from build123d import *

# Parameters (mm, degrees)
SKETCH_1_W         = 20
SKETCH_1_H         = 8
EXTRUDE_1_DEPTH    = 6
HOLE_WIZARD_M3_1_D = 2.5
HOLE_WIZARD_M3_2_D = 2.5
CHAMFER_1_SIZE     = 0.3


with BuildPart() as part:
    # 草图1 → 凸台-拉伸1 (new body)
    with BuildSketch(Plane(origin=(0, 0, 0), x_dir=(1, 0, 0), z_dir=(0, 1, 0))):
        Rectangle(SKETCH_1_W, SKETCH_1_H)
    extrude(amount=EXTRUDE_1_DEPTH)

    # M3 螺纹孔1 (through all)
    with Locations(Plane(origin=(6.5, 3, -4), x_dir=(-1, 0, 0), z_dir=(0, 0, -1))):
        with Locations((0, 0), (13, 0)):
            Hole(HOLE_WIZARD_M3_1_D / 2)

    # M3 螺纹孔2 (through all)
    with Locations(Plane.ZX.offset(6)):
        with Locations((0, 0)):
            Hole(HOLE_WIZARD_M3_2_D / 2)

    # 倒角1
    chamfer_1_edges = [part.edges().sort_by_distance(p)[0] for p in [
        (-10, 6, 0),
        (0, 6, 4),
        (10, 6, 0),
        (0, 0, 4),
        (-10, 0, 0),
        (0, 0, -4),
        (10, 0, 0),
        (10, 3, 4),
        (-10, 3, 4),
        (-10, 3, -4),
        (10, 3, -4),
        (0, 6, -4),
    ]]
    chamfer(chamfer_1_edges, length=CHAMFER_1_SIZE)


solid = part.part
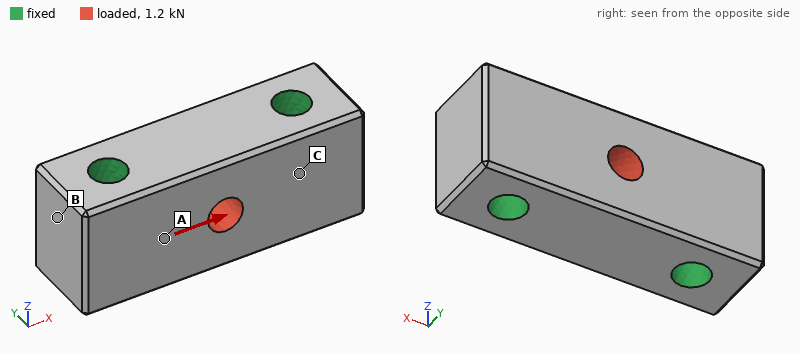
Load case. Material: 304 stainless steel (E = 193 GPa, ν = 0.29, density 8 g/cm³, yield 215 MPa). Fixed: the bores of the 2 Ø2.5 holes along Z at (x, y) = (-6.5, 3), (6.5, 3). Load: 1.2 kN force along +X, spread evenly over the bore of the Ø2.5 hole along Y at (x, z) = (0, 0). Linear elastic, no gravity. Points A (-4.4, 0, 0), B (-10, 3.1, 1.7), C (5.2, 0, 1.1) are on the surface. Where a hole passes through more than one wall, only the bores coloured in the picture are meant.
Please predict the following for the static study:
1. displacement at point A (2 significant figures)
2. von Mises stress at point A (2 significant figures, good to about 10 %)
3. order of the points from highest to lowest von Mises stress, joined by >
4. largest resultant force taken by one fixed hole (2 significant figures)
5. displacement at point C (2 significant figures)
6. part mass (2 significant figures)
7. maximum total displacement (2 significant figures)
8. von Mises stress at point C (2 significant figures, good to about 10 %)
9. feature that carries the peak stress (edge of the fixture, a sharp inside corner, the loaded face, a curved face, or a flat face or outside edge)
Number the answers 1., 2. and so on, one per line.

1. 0.19 µm
2. 12 MPa
3. A > C > B
4. 600 N
5. 0.14 µm
6. 6.8 g
7. 0.52 µm
8. 8.5 MPa
9. the loaded face
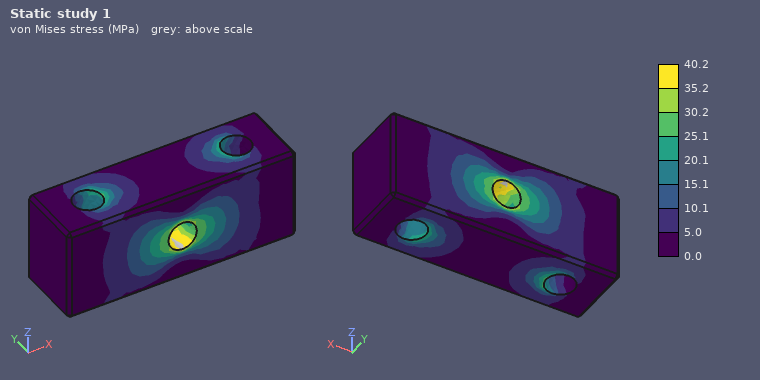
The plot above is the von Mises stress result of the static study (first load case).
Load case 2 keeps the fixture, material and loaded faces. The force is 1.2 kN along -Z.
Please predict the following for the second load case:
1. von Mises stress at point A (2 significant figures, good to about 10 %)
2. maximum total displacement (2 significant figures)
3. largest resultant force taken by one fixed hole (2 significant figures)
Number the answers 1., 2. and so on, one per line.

1. 22 MPa
2. 1.3 µm
3. 600 N
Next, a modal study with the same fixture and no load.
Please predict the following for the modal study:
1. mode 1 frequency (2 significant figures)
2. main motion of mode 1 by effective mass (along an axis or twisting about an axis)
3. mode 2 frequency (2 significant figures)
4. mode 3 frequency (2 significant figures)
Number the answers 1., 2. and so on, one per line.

1. 96 kHz
2. along Y
3. 120 kHz
4. 120 kHz
